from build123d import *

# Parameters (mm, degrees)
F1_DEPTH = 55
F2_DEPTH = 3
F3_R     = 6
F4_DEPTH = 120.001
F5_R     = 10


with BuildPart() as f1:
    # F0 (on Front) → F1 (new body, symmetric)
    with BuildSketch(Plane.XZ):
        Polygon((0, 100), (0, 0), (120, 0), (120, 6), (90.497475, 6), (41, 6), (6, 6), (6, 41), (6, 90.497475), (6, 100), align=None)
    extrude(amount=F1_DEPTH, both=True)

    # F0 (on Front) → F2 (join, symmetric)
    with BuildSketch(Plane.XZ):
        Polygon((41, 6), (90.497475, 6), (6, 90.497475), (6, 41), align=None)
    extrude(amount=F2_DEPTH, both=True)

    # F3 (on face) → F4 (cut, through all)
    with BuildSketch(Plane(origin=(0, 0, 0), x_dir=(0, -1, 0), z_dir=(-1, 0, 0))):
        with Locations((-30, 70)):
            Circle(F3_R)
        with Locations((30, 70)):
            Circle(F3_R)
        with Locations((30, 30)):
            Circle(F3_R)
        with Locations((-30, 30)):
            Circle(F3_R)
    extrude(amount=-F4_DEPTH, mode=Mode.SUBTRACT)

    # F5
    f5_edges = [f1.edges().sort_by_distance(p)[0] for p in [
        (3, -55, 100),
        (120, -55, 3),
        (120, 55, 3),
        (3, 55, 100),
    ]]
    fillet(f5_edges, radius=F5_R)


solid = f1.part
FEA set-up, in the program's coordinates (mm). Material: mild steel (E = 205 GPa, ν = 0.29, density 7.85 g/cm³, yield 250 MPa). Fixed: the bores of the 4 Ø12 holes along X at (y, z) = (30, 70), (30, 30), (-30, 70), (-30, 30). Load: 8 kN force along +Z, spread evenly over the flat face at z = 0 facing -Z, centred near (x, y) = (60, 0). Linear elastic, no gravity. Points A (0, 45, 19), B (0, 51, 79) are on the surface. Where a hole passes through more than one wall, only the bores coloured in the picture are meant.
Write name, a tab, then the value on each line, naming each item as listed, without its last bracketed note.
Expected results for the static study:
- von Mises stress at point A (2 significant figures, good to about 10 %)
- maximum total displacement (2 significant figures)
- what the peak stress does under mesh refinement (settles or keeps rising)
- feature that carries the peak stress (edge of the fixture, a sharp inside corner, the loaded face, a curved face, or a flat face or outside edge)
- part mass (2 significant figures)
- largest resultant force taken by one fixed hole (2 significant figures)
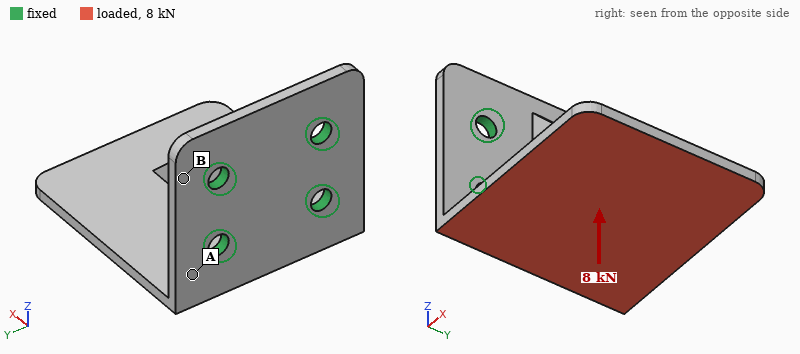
von Mises stress at point A	100 MPa
maximum total displacement	0.45 mm
what the peak stress does under mesh refinement	keeps rising
feature that carries the peak stress	edge of the fixture
part mass	1.2 kg
largest resultant force taken by one fixed hole	4.3 kN
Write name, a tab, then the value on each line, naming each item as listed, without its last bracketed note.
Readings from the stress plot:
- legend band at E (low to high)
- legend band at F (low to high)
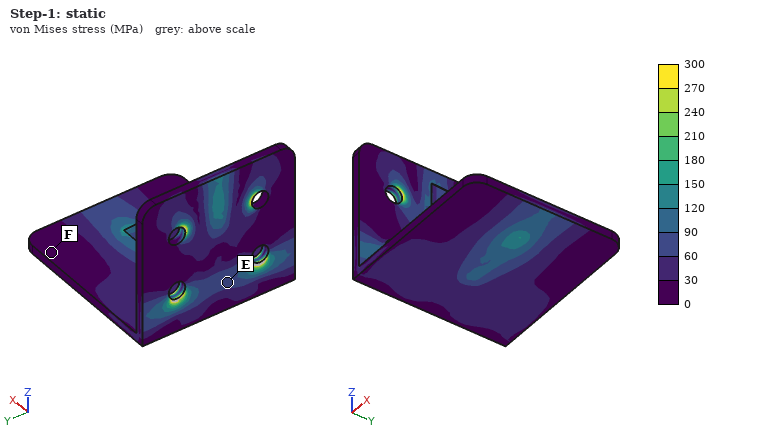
legend band at E	60 to 90 MPa
legend band at F	0 to 30 MPa
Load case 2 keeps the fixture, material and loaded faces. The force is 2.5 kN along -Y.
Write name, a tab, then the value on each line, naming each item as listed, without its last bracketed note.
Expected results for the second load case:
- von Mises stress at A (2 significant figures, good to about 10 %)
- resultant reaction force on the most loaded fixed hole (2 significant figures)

von Mises stress at A	44 MPa
resultant reaction force on the most loaded fixed hole	2.6 kN
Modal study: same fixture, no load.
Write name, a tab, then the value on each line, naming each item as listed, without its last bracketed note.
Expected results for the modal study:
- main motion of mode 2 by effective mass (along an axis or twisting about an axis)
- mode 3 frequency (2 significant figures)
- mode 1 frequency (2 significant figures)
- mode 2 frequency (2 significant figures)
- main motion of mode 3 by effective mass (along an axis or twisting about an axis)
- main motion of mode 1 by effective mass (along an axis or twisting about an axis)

main motion of mode 2 by effective mass	along Z
mode 3 frequency	1100 Hz
mode 1 frequency	870 Hz
mode 2 frequency	1100 Hz
main motion of mode 3 by effective mass	along Y
main motion of mode 1 by effective mass	along Y
